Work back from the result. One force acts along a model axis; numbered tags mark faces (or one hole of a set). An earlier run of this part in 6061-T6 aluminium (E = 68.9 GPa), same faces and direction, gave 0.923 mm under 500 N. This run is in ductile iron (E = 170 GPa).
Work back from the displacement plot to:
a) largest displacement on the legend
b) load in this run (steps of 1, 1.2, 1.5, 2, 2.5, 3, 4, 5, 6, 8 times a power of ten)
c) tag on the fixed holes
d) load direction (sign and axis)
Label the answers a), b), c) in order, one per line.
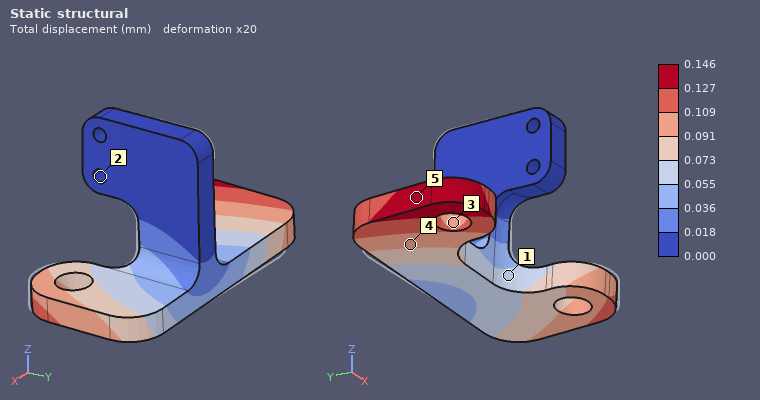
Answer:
a) 0.146 mm
b) 200 N
c) 2
d) -X
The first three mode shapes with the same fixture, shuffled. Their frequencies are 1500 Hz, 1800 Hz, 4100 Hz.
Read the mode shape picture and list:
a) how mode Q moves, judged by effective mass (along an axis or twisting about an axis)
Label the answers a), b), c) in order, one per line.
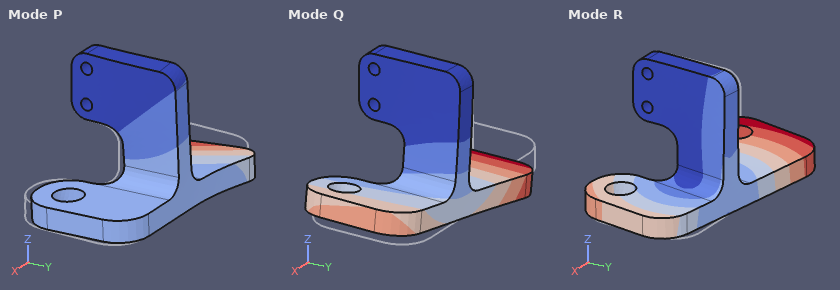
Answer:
a) along X
